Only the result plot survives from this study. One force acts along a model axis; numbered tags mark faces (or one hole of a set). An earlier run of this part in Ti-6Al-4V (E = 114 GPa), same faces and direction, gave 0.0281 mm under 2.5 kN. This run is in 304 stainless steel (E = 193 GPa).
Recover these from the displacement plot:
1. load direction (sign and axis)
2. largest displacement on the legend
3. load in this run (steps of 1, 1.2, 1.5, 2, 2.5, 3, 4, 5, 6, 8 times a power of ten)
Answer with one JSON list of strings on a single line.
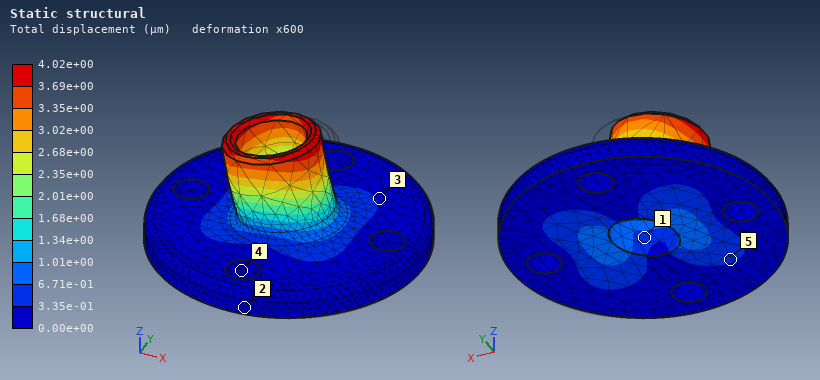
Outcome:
["-X", "4.02e+00 µm", "600 N"]
